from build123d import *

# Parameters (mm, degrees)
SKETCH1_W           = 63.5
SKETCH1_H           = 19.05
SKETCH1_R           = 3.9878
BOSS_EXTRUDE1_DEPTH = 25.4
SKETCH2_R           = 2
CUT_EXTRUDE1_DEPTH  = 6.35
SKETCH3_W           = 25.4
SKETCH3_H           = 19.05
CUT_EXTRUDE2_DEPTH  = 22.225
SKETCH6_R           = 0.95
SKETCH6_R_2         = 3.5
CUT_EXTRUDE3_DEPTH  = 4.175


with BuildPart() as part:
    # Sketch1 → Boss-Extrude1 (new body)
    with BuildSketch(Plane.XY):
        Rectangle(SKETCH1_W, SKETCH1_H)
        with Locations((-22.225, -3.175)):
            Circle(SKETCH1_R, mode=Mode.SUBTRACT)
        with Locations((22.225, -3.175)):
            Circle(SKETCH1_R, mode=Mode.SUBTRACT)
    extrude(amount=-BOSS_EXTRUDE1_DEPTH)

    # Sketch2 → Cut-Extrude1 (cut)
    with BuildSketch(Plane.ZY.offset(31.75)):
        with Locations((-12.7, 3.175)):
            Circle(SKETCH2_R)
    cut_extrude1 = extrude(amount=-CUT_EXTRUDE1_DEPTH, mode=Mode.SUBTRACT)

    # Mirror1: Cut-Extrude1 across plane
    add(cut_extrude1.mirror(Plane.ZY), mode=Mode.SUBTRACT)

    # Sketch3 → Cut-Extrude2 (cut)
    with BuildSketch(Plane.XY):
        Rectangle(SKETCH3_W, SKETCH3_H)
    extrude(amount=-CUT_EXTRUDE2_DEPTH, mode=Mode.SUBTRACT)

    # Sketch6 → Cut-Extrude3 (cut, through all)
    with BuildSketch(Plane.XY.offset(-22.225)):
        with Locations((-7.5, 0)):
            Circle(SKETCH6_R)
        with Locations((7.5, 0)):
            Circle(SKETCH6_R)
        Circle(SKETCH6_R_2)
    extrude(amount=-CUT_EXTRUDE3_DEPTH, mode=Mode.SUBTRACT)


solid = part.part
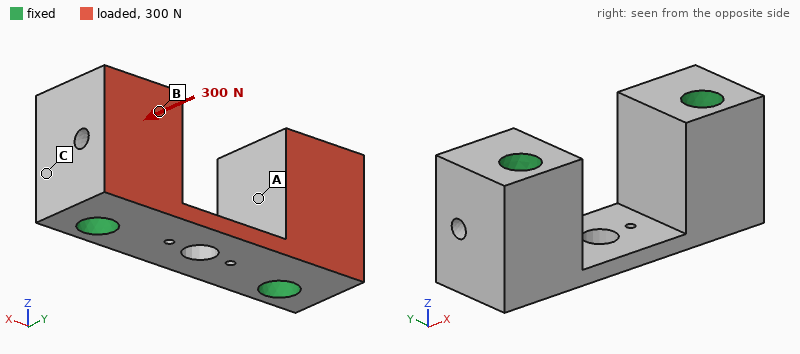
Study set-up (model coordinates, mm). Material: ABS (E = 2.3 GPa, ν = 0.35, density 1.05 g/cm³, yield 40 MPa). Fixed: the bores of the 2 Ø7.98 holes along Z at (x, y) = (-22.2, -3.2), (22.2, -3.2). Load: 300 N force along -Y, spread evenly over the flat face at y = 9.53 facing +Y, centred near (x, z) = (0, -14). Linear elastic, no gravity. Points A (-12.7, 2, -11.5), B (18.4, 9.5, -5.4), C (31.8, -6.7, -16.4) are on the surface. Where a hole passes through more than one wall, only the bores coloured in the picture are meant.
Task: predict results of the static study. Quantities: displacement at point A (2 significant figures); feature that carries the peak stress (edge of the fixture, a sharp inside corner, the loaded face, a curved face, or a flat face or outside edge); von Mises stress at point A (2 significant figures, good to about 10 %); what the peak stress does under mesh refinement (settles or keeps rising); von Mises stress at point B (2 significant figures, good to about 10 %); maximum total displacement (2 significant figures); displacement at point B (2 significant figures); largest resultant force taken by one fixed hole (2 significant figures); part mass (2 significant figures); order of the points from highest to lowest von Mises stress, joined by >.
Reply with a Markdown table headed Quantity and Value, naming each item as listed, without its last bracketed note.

| Quantity | Value |
|---|---|
| displacement at point A | 1.2 µm |
| feature that carries the peak stress | edge of the fixture |
| von Mises stress at point A | 0.17 MPa |
| what the peak stress does under mesh refinement | keeps rising |
| von Mises stress at point B | 0.36 MPa |
| maximum total displacement | 6.2 µm |
| displacement at point B | 1.6 µm |
| largest resultant force taken by one fixed hole | 150 N |
| part mass | 18 g |
| order of the points from highest to lowest von Mises stress, joined by > | B > A > C |
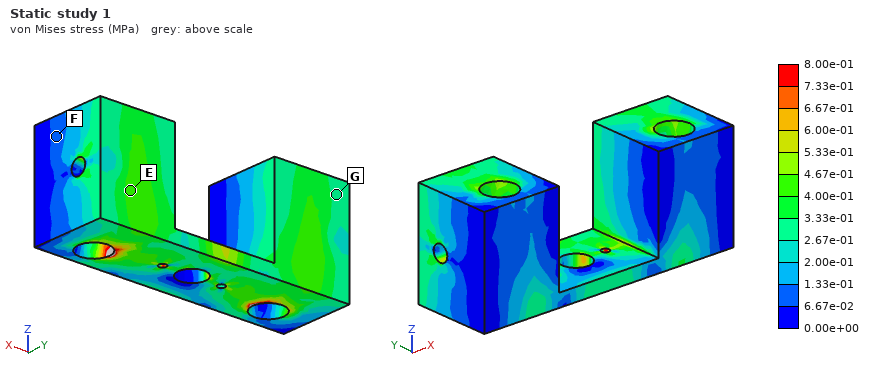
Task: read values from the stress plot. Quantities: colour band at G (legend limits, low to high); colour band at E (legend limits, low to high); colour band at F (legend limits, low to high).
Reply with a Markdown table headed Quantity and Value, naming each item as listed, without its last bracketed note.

| Quantity | Value |
|---|---|
| colour band at G | 2.67e-01 to 3.33e-01 MPa |
| colour band at E | 4.00e-01 to 4.67e-01 MPa |
| colour band at F | 6.67e-02 to 1.33e-01 MPa |
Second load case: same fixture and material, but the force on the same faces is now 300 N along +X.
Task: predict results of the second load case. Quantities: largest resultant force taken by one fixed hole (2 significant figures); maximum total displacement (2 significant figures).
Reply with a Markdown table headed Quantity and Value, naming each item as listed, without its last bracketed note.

| Quantity | Value |
|---|---|
| largest resultant force taken by one fixed hole | 150 N |
| maximum total displacement | 11 µm |
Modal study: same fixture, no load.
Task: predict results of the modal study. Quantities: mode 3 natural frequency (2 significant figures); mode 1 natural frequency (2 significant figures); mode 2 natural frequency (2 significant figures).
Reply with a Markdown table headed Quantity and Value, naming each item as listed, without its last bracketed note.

| Quantity | Value |
|---|---|
| mode 3 natural frequency | 10 kHz |
| mode 1 natural frequency | 5600 Hz |
| mode 2 natural frequency | 7100 Hz |
